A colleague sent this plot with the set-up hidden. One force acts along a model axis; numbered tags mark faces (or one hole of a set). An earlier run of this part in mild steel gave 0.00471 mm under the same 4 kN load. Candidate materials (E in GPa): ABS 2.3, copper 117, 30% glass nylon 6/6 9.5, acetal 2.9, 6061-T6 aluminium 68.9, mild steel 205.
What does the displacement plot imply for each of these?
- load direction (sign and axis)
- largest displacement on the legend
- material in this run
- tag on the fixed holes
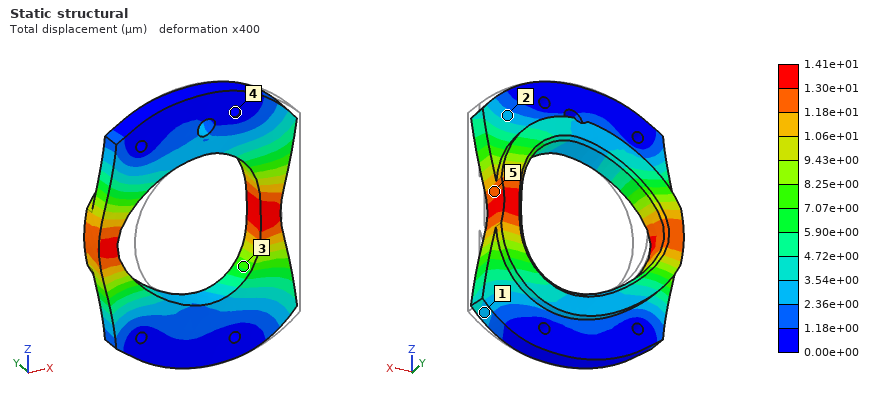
-X
1.41e+01 µm
6061-T6 aluminium
4
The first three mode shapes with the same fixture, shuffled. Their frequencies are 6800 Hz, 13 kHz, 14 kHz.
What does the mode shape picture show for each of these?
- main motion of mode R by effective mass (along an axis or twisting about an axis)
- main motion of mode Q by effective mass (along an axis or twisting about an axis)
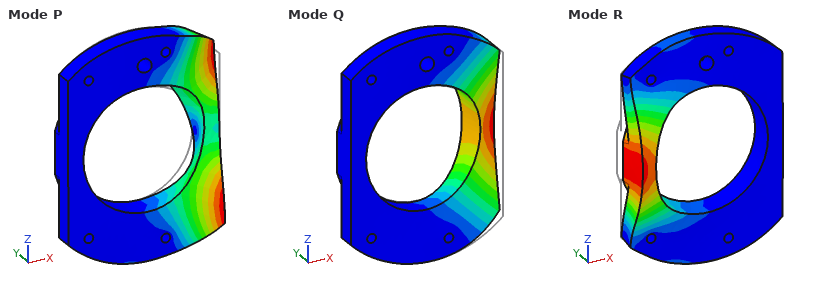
along Y
along Y
